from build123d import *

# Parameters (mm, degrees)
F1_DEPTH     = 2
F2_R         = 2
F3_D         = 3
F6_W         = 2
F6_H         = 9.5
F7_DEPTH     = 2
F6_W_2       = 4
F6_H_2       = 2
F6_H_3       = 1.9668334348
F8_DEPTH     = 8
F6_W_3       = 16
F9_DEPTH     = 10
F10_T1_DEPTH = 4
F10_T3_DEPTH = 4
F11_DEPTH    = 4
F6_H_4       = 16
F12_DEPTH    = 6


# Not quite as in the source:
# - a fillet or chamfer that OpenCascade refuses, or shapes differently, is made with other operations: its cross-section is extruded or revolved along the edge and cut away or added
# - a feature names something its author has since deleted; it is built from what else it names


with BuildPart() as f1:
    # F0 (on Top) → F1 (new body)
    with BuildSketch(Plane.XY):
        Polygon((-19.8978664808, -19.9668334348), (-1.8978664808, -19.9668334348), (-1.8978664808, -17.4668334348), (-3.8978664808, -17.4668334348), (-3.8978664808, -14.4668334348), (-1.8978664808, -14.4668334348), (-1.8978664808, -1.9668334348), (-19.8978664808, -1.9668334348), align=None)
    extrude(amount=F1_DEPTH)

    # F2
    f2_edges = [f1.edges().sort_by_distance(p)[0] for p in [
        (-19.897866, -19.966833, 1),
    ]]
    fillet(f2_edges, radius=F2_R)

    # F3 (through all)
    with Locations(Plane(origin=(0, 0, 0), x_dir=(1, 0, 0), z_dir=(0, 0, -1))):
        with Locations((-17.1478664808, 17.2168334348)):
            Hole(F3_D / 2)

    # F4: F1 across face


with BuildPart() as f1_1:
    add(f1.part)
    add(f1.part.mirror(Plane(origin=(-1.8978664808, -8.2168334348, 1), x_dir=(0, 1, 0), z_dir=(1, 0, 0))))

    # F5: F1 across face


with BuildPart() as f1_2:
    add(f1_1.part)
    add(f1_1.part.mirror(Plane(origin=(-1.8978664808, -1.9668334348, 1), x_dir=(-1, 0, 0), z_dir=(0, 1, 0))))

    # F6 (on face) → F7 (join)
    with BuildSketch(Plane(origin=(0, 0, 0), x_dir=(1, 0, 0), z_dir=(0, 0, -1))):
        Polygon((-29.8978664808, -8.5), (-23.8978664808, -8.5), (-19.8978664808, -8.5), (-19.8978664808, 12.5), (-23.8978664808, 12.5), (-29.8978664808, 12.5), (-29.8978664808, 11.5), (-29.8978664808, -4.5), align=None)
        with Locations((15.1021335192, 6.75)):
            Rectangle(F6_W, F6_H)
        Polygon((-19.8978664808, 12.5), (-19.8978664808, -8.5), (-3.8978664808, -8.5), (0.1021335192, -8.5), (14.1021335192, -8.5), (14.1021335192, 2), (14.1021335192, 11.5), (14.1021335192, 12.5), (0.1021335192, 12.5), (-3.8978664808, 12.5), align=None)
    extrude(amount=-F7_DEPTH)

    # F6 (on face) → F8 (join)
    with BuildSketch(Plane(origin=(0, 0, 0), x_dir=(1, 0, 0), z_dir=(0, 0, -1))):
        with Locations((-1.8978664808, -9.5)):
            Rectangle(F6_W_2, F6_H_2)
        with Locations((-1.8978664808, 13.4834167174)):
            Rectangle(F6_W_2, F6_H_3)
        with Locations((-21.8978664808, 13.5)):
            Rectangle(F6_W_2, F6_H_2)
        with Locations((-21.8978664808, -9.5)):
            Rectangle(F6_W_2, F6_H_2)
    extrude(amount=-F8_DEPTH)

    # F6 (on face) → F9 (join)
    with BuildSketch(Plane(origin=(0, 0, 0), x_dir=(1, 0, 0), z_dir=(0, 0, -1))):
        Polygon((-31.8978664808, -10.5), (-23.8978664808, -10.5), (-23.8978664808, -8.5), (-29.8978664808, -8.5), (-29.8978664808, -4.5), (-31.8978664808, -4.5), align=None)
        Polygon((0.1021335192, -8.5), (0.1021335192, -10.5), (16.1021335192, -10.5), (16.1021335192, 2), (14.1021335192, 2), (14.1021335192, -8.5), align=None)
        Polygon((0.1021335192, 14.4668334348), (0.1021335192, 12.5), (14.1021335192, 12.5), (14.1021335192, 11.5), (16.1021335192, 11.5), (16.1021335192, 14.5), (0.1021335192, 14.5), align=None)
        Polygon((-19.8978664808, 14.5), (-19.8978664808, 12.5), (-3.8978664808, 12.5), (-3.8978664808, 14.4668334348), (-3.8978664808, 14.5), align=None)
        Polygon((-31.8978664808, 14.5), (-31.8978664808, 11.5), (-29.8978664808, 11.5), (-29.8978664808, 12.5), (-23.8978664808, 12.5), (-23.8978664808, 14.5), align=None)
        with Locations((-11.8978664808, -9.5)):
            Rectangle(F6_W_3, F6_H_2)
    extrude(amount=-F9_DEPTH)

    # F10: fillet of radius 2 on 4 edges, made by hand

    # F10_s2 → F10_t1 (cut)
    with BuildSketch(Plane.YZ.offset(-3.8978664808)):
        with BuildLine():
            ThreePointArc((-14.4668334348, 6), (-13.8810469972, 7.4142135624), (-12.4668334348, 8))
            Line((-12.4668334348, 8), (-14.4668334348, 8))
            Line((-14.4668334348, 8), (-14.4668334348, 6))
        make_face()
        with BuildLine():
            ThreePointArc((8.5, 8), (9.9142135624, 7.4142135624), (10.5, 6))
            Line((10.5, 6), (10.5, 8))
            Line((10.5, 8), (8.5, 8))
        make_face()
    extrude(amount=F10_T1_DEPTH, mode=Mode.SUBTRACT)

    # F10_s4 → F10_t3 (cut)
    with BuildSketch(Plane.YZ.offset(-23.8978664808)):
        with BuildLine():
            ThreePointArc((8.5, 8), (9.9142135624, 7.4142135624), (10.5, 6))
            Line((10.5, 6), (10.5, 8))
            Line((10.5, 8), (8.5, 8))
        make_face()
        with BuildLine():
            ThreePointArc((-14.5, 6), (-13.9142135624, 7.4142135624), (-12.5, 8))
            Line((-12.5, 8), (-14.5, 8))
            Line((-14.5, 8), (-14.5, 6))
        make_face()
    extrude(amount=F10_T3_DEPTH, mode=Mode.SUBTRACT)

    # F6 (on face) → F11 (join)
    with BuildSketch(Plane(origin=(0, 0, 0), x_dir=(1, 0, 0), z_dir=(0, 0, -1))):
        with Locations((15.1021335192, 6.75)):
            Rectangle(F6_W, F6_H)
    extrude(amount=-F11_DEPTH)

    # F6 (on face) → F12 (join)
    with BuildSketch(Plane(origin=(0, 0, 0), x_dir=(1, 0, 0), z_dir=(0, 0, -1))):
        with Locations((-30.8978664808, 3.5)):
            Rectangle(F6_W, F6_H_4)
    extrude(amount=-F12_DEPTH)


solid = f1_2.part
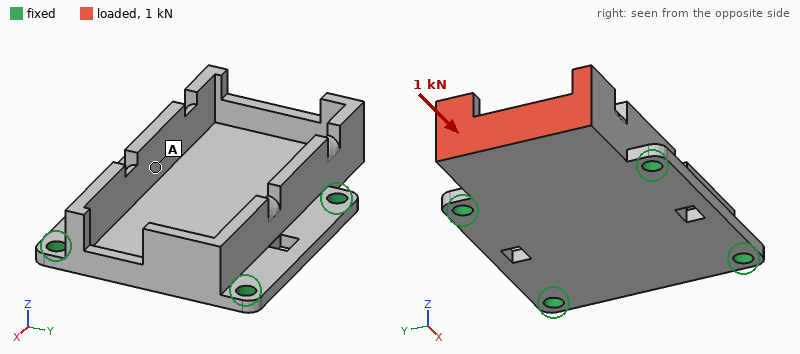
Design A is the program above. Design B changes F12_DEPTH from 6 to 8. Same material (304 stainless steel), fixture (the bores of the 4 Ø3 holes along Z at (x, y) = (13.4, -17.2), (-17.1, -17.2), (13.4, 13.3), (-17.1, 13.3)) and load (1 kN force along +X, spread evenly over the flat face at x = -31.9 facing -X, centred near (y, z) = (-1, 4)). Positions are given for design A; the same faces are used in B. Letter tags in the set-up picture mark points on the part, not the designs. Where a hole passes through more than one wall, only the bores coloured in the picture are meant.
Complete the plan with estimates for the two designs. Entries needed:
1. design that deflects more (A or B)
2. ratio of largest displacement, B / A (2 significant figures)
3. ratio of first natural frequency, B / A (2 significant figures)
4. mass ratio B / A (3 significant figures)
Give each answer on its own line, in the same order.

B
1.4
1.0
1.01
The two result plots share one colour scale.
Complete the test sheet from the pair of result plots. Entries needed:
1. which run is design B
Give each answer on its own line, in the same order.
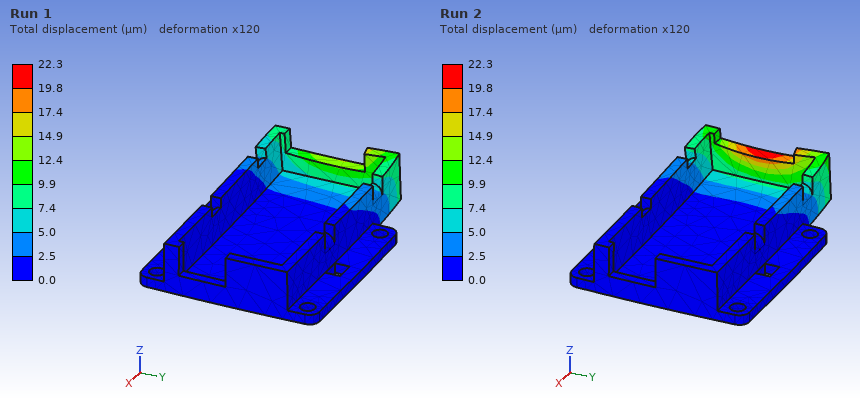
Run 2
